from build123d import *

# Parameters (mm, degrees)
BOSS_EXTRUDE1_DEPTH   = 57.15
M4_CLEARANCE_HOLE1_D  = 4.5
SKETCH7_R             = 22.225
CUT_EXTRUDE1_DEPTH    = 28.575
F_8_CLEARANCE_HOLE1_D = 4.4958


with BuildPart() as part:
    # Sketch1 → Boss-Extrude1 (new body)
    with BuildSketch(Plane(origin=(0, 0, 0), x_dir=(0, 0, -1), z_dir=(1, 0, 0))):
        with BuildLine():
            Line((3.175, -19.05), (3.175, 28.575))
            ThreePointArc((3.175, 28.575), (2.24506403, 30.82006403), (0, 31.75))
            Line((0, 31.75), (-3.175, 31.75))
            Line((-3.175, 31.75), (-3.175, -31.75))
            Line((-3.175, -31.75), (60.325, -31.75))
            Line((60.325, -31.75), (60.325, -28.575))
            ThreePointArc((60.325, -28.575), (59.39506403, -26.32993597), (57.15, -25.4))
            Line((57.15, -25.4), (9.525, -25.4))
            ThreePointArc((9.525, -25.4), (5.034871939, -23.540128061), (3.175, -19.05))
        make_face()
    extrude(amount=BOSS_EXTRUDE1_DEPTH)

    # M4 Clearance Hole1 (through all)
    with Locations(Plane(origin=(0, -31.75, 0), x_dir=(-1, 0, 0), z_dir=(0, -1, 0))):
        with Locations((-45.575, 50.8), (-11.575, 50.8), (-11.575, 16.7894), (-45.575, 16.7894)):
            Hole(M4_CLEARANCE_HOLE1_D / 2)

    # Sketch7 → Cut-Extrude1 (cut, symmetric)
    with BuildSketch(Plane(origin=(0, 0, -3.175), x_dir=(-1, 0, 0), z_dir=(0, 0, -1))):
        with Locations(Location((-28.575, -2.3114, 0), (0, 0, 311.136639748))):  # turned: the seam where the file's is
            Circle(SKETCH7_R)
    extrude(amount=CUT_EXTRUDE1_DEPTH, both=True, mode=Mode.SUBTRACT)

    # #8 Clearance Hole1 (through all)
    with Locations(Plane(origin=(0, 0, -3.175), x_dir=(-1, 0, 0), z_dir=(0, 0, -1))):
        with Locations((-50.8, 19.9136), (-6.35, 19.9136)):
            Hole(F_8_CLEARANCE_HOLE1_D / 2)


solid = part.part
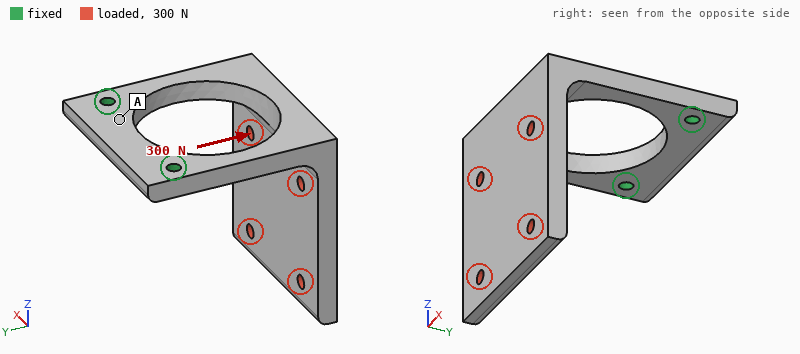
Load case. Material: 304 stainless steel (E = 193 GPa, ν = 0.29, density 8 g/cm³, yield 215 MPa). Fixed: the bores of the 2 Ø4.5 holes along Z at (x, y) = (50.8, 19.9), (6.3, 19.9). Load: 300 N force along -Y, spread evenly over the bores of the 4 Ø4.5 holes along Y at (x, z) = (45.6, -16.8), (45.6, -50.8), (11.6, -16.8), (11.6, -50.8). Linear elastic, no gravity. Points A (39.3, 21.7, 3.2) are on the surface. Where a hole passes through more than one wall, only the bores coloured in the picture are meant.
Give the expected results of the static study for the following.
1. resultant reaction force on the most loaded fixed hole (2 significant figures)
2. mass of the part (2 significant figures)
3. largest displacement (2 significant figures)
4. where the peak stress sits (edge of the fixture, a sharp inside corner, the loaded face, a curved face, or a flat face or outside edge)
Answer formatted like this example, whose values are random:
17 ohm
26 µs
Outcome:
160 N
270 g
0.45 mm
a curved face
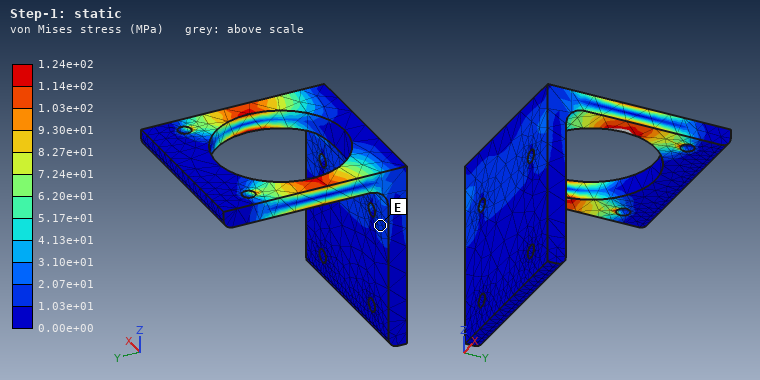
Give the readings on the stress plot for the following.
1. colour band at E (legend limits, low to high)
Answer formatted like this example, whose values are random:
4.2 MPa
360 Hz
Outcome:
1.03e+01 to 2.07e+01 MPa
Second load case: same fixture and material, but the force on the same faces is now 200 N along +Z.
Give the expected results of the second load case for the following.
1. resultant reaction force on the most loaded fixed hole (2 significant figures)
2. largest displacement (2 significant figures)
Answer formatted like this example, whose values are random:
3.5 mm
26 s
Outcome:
100 N
0.22 mm
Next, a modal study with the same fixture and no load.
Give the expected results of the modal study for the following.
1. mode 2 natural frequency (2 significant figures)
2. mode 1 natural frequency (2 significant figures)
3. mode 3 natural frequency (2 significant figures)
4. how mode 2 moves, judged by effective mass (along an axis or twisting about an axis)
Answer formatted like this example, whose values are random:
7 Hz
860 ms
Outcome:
770 Hz
340 Hz
1300 Hz
along X
